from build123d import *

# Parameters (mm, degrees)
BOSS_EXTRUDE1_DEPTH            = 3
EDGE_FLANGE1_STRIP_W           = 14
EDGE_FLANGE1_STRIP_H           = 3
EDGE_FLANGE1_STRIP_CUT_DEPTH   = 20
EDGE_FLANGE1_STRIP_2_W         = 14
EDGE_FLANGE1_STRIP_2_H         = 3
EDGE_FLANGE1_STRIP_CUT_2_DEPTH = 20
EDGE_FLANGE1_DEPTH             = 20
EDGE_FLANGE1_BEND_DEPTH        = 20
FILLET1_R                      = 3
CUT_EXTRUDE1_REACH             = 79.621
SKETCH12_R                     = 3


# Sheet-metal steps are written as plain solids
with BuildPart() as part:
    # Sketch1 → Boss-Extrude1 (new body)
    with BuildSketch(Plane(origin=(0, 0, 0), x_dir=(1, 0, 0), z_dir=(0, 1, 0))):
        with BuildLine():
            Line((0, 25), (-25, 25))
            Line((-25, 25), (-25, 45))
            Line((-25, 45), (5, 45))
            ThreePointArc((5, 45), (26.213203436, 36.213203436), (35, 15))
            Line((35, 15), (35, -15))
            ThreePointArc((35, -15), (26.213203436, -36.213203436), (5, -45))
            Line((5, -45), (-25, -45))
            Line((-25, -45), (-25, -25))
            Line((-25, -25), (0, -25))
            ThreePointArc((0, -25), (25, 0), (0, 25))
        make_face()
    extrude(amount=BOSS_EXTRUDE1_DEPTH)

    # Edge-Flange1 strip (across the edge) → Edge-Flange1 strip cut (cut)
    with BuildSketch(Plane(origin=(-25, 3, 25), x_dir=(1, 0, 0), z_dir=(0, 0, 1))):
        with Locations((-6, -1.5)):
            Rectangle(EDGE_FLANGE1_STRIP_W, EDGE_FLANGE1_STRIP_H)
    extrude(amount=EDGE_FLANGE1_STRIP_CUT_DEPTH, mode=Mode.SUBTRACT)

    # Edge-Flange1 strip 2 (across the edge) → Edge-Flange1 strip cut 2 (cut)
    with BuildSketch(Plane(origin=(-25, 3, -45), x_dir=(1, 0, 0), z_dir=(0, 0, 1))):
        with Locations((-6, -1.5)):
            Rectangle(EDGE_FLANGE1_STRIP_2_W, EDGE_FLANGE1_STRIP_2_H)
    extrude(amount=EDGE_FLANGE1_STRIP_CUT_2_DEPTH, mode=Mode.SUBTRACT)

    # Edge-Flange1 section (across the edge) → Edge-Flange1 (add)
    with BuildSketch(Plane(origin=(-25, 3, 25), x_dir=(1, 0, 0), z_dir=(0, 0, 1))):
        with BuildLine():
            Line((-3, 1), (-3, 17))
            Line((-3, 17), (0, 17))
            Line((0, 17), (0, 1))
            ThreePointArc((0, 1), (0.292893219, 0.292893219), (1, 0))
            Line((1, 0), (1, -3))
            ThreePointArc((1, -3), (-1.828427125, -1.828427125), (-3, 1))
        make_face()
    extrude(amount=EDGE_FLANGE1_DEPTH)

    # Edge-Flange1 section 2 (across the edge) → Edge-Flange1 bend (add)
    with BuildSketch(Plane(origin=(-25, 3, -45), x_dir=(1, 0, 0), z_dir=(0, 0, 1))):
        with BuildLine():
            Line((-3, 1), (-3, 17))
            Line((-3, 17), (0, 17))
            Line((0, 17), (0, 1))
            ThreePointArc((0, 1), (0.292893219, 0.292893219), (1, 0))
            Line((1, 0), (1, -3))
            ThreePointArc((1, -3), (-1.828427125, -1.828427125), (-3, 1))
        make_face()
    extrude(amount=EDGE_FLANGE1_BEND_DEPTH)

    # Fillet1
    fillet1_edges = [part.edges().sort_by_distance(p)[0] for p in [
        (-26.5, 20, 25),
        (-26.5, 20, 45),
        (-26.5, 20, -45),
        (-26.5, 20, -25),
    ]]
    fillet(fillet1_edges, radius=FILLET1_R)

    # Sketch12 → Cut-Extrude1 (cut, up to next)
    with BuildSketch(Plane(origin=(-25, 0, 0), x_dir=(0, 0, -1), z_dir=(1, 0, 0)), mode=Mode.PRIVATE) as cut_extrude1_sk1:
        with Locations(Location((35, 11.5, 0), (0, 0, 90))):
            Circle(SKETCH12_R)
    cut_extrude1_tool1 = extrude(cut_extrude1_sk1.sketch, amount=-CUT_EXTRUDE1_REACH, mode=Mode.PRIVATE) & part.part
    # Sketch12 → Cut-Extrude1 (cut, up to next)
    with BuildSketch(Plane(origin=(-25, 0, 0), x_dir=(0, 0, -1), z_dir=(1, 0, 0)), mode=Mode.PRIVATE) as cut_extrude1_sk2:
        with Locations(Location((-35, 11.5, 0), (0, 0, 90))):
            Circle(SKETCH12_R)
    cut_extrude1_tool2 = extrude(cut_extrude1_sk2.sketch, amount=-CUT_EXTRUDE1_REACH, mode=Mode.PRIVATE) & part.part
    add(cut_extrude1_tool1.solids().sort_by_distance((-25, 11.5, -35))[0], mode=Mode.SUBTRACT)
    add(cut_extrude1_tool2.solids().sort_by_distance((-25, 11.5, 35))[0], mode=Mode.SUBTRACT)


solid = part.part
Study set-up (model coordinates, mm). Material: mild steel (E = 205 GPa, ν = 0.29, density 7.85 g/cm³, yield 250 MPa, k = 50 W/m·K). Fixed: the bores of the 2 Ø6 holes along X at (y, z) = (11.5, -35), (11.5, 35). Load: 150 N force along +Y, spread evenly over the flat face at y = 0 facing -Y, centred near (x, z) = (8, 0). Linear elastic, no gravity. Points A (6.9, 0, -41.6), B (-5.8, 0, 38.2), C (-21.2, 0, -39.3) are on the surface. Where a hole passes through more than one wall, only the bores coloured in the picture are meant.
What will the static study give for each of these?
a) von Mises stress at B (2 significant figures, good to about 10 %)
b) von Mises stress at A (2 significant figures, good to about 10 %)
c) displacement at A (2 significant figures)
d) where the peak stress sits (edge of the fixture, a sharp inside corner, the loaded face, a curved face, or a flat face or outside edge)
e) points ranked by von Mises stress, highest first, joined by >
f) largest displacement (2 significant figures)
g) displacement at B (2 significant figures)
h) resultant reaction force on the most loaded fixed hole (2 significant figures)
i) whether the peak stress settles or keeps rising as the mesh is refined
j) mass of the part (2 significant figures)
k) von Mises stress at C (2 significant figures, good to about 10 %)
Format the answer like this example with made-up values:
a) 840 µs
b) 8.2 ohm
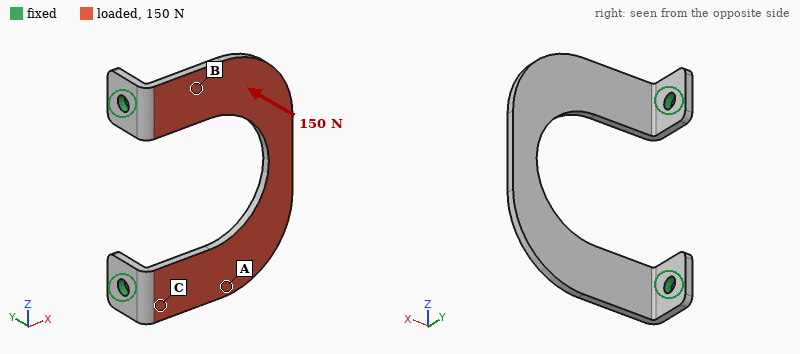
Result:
a) 40 MPa
b) 20 MPa
c) 0.17 mm
d) edge of the fixture
e) C > B > A
f) 0.42 mm
g) 0.091 mm
h) 75 N
i) keeps rising
j) 82 g
k) 68 MPa
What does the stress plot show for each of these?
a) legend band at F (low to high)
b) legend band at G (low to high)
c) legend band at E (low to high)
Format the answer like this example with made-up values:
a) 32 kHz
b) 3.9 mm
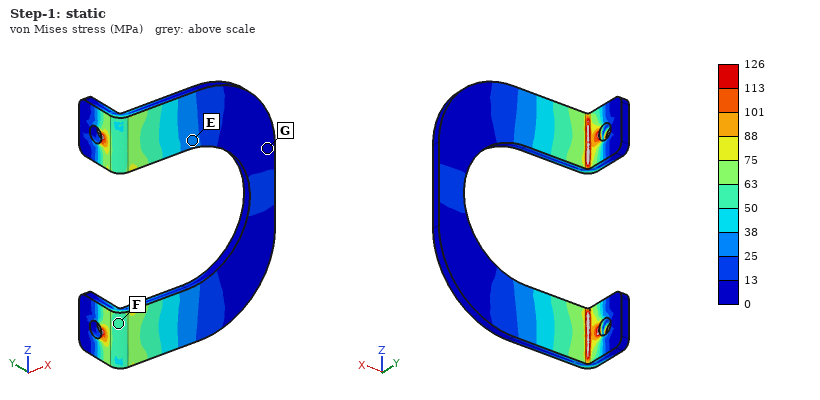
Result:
a) 50 to 63 MPa
b) 0 to 13 MPa
c) 25 to 38 MPa
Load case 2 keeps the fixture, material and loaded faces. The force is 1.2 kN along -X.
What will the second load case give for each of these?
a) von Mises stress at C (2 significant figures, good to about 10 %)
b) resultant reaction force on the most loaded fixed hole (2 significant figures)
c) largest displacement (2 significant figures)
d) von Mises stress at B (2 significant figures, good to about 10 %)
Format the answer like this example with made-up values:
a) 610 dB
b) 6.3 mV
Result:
a) 37 MPa
b) 600 N
c) 0.33 mm
d) 27 MPa
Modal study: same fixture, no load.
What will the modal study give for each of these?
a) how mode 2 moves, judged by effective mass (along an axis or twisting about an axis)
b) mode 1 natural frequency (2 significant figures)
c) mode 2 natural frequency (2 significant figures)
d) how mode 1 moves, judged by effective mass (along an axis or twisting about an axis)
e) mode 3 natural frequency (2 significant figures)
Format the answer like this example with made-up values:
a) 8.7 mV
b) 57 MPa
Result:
a) twisting about X
b) 460 Hz
c) 1100 Hz
d) along Y
e) 2500 Hz
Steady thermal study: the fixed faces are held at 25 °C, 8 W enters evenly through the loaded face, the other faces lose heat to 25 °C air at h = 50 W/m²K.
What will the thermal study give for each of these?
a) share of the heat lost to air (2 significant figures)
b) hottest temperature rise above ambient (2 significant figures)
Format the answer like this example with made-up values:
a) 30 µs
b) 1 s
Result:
a) 51 %
b) 27 K
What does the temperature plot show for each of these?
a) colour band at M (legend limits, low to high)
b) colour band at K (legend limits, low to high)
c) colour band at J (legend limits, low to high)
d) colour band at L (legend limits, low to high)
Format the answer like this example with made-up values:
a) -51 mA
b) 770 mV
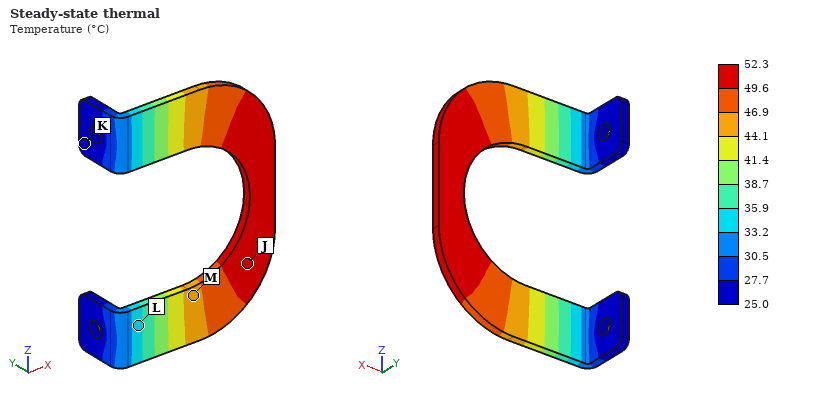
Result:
a) 44.1 to 46.9 °C
b) 25.0 to 27.7 °C
c) 49.6 to 52.3 °C
d) 33.2 to 35.9 °C
